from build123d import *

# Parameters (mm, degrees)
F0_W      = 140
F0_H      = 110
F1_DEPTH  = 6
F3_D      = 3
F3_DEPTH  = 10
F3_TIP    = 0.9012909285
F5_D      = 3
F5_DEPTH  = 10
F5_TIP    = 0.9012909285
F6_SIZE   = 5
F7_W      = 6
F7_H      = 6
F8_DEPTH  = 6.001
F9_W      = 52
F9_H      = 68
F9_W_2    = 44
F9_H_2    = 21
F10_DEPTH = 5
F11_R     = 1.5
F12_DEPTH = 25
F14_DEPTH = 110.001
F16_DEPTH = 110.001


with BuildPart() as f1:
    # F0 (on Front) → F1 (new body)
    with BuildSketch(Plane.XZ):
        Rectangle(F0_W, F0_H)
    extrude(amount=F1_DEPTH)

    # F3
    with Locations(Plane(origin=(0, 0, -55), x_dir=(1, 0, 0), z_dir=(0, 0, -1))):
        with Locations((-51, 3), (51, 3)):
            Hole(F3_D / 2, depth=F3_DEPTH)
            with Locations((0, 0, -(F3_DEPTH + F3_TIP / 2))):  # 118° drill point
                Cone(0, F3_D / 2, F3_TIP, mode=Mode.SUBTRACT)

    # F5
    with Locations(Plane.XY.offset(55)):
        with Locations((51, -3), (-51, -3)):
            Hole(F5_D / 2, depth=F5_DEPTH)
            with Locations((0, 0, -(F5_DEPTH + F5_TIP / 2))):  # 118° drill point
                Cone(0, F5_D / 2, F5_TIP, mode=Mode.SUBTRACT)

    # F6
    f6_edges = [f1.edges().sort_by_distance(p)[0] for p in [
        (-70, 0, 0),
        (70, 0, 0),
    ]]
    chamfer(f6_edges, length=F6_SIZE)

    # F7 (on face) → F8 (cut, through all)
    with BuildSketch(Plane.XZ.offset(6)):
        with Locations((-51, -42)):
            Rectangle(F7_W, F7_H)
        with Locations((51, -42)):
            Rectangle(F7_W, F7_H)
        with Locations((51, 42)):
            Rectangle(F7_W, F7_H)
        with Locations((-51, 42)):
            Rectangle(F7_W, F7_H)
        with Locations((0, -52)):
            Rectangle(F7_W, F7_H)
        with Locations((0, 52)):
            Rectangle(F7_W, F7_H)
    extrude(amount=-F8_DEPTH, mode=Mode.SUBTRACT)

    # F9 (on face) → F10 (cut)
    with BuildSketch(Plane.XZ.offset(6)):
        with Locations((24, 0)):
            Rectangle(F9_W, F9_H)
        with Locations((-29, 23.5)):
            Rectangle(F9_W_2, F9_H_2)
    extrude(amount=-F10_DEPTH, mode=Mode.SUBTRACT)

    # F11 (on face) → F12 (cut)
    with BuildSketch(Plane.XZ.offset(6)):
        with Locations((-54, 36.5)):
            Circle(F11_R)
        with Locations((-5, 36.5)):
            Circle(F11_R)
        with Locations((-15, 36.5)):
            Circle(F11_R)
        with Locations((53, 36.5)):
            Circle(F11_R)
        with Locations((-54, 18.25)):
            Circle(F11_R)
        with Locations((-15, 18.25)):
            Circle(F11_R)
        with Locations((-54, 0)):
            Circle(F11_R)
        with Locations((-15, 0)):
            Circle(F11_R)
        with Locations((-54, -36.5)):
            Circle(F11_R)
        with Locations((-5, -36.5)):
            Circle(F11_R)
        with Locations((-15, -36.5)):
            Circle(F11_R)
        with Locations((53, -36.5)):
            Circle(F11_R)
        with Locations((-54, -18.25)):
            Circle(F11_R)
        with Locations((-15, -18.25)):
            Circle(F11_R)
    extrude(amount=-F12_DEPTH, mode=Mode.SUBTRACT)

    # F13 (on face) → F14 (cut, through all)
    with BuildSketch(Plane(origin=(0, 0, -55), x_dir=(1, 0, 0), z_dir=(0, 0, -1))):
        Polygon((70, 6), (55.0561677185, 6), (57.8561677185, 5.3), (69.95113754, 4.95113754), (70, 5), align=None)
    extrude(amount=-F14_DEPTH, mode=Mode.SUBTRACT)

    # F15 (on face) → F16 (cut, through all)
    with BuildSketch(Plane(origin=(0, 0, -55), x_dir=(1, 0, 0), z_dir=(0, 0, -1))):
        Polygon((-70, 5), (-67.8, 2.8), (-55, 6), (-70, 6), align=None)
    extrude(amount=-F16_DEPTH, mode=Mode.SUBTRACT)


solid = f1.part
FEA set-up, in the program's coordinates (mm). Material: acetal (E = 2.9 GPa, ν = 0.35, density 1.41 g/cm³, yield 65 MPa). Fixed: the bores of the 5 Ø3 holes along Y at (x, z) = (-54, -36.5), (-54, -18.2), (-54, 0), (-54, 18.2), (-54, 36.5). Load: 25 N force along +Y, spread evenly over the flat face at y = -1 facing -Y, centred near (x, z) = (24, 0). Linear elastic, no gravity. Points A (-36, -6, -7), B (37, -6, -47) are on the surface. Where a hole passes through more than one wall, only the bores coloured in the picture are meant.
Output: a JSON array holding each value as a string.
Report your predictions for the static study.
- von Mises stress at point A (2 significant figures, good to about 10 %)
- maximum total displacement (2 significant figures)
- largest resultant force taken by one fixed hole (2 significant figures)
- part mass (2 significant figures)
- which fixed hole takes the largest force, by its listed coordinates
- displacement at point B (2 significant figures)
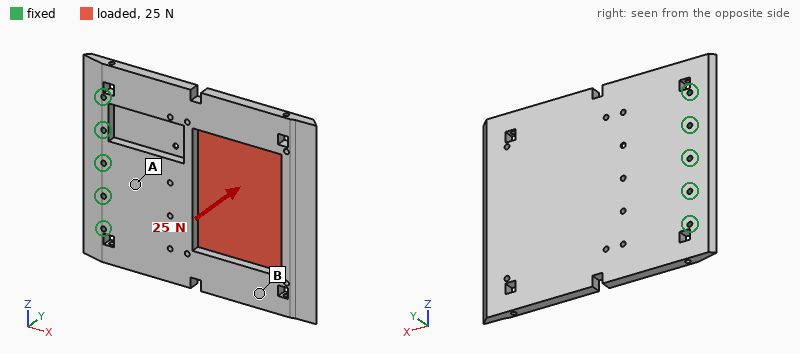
["2.5 MPa", "2.0 mm", "35 N", "86 g", "(-54, 18.2)", "1.2 mm"]
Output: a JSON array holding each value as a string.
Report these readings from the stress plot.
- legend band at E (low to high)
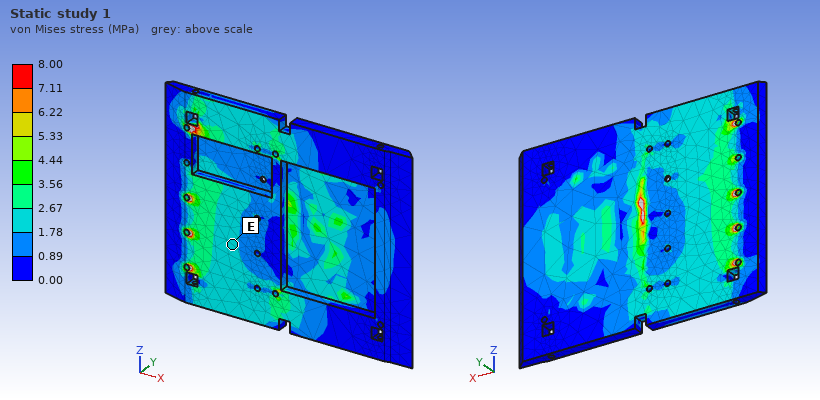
["1.78 to 2.67 MPa"]
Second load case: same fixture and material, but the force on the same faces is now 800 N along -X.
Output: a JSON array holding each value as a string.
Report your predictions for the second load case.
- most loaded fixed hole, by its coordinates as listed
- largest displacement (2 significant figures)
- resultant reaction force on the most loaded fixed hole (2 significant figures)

["(-54, 36.5)", "1.8 mm", "220 N"]
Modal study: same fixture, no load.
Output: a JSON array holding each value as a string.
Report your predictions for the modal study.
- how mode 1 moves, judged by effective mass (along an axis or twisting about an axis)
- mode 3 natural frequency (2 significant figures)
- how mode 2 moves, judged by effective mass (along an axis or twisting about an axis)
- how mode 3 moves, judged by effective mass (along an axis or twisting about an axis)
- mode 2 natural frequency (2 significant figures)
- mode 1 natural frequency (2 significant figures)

["along Y", "460 Hz", "twisting about X", "along Y", "180 Hz", "92 Hz"]
